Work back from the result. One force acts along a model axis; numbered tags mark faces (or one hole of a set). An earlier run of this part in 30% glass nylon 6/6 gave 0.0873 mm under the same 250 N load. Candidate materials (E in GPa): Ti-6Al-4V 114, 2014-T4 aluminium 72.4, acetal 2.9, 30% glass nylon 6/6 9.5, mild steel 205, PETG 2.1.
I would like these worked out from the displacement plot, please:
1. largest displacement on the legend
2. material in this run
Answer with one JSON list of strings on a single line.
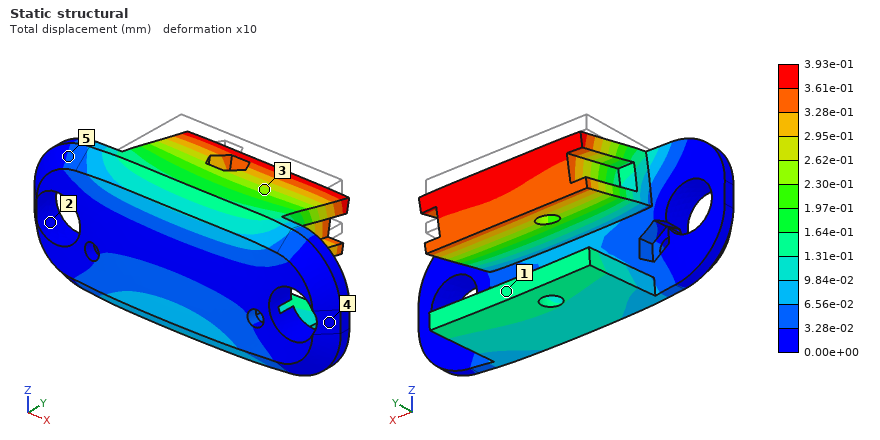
["3.93e-01 mm", "PETG"]
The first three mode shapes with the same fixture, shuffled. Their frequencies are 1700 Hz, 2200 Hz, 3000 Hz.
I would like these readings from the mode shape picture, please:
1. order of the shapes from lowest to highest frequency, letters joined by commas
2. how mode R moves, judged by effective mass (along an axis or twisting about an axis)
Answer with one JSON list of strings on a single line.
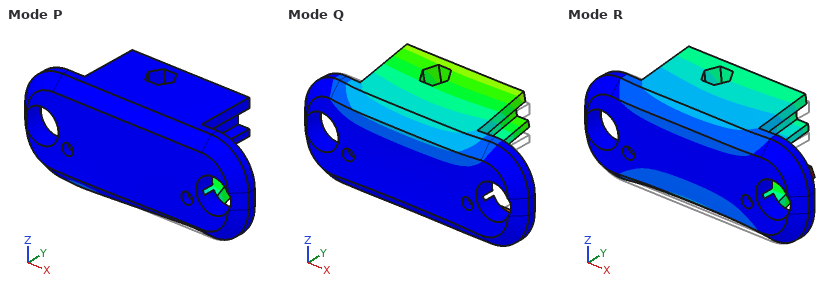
["R, Q, P", "along Z"]
